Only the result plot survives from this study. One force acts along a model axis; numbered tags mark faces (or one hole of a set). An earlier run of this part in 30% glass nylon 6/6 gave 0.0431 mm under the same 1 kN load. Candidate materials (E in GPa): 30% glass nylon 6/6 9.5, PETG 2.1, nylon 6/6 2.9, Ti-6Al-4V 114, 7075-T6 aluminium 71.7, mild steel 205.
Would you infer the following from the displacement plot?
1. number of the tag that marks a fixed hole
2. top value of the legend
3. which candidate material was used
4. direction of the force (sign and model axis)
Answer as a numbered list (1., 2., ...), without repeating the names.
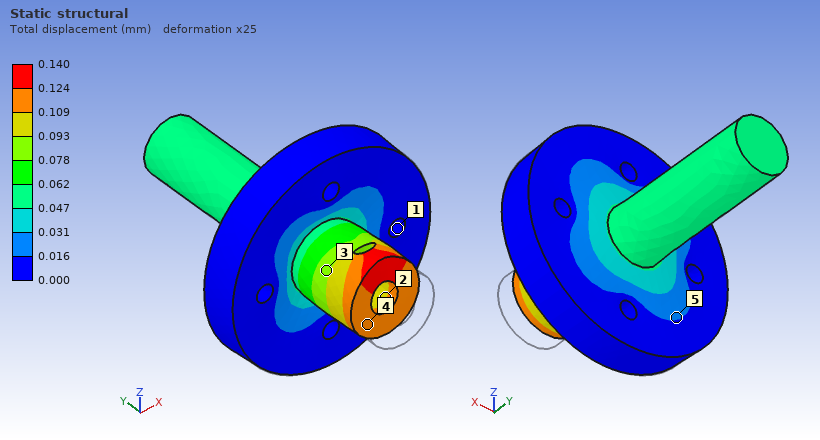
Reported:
1. 1
2. 0.140 mm
3. nylon 6/6
4. +Y
